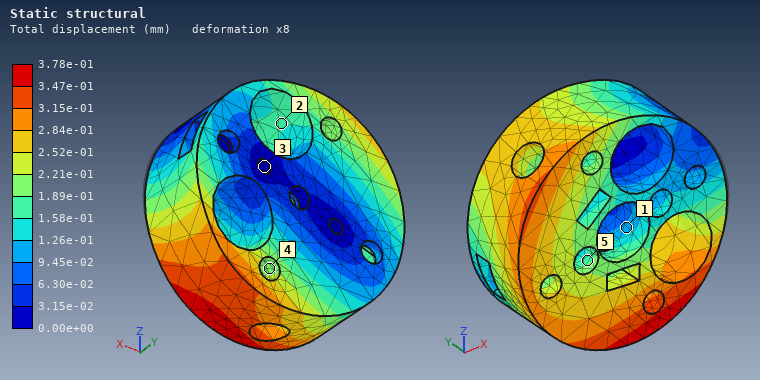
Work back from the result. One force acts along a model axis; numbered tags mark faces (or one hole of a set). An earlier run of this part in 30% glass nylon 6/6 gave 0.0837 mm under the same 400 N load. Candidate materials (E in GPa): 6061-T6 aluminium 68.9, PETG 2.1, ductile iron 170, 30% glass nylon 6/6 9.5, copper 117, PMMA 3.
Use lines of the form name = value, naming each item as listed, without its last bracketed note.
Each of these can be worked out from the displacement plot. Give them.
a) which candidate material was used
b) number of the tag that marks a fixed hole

which candidate material was used = PETG
number of the tag that marks a fixed hole = 3
